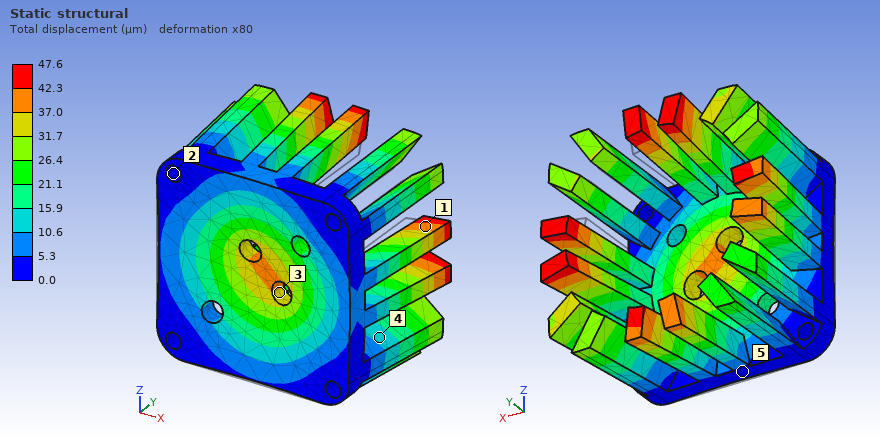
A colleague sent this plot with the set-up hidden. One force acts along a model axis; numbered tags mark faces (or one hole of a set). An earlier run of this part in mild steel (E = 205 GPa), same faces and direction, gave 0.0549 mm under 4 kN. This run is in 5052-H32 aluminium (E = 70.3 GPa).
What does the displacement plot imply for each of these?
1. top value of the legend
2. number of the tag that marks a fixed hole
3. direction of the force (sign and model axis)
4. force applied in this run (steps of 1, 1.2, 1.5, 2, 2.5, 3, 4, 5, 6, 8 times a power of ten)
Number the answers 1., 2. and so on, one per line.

1. 47.6 µm
2. 2
3. +Y
4. 1.2 kN
